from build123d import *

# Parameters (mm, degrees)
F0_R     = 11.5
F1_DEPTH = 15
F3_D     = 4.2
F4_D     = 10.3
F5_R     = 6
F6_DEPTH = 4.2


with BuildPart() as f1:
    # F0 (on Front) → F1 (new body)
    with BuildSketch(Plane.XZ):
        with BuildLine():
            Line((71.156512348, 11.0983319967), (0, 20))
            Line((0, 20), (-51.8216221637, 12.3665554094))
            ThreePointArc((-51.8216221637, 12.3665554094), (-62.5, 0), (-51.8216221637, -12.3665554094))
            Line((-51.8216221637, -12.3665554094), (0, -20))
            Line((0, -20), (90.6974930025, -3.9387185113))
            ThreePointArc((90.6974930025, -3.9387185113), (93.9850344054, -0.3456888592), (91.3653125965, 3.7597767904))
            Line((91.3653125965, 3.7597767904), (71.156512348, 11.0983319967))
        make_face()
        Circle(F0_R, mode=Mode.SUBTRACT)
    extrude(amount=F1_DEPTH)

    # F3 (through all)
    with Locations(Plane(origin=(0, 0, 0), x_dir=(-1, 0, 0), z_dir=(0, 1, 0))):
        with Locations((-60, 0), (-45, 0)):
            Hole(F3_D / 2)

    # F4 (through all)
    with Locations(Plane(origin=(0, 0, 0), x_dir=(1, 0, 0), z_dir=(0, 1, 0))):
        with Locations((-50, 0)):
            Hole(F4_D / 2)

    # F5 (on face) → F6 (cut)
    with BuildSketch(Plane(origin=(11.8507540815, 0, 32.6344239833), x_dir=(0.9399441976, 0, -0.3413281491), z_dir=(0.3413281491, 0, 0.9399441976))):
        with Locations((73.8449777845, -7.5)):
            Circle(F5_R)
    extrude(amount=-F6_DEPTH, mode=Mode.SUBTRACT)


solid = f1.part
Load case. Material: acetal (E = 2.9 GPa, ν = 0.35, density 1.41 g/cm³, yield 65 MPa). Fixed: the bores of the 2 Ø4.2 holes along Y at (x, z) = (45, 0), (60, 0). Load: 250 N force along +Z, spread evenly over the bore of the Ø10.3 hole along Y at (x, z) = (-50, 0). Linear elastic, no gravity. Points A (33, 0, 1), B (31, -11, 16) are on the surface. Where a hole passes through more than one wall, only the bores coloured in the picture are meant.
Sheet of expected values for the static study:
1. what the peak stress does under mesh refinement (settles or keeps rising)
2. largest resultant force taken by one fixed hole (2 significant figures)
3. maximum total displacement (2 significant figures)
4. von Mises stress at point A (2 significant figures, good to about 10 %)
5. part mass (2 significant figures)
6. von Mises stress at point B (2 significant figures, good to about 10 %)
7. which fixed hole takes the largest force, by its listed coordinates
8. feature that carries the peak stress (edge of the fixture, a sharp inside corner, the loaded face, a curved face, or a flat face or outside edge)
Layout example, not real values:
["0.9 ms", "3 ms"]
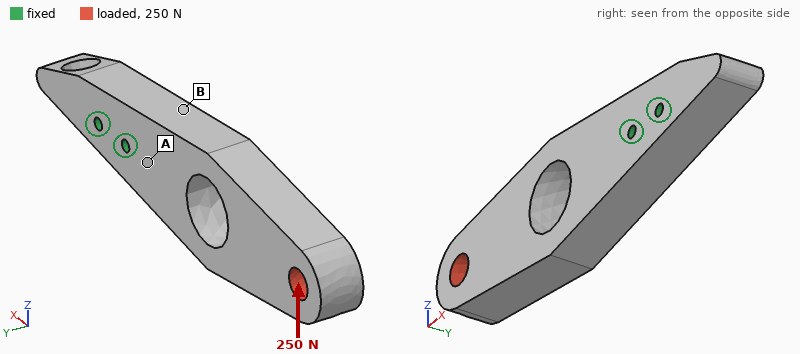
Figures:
["keeps rising", "1.4 kN", "1.5 mm", "2.7 MPa", "78 g", "8.8 MPa", "(45, 0)", "edge of the fixture"]
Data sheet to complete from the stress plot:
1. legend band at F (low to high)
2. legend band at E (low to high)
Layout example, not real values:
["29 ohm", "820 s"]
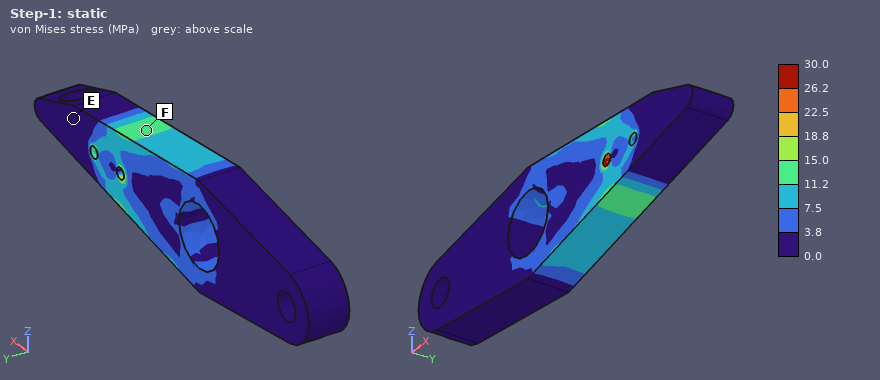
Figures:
["11.2 to 15.0 MPa", "0.0 to 3.8 MPa"]
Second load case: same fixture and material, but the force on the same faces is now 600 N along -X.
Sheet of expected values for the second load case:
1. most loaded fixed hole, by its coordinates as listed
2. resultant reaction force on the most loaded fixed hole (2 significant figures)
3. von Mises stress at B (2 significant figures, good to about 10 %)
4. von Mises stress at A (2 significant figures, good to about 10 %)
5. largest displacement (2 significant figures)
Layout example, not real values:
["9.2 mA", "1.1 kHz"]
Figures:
["(45, 0)", "450 N", "1.4 MPa", "1.3 MPa", "83 µm"]
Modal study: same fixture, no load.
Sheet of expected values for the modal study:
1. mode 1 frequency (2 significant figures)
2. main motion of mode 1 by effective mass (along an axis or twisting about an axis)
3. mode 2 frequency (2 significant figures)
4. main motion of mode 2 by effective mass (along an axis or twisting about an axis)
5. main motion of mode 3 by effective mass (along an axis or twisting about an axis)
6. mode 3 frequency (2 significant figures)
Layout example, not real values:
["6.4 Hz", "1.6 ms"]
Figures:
["300 Hz", "along Y", "460 Hz", "along Z", "twisting about X", "1400 Hz"]
